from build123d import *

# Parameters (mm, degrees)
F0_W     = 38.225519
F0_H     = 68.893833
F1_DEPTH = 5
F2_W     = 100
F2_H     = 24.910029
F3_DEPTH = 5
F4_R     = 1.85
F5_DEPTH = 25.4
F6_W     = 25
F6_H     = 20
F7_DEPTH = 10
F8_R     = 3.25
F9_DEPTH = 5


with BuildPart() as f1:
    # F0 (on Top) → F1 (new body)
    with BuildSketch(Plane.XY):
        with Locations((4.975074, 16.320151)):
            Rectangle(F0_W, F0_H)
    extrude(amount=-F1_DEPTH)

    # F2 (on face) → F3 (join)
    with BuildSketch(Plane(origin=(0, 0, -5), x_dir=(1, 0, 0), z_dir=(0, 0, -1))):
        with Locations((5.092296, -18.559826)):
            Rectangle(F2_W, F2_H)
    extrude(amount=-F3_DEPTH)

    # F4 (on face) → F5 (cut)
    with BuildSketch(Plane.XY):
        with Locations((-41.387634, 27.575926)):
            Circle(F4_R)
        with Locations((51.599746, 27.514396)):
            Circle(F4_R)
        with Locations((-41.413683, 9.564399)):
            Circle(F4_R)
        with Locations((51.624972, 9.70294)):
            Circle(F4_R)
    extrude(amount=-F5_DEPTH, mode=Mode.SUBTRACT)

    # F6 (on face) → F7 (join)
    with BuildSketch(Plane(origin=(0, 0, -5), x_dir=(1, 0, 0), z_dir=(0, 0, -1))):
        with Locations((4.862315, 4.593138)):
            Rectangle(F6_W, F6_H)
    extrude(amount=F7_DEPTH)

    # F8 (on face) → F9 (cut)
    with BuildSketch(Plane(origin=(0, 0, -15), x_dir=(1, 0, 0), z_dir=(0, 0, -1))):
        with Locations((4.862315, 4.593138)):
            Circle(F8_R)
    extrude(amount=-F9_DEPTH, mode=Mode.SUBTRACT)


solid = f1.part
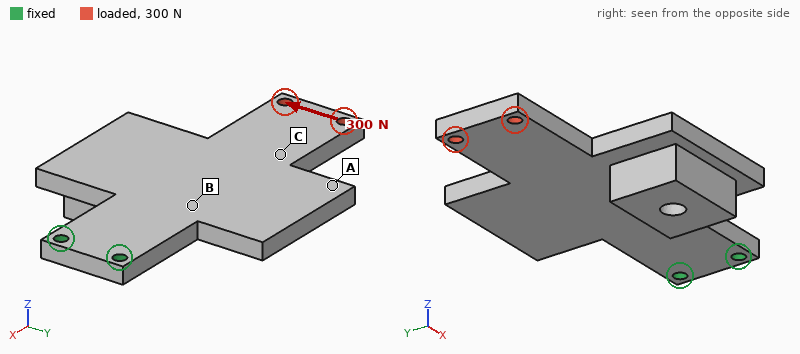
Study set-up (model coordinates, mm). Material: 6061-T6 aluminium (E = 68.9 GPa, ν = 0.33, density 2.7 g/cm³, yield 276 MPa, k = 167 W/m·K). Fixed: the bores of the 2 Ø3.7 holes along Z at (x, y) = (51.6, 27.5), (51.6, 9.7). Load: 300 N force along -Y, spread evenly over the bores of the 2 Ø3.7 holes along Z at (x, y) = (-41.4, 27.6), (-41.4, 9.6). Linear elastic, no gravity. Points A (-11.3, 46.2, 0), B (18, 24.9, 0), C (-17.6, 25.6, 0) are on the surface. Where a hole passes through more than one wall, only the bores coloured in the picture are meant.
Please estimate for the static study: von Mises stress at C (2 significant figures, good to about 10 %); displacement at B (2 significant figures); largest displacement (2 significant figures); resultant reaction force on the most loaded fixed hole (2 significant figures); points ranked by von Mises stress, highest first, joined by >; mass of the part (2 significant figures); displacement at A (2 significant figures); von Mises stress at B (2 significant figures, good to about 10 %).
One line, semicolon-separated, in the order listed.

7.7 MPa; 0.036 mm; 0.17 mm; 1.5 kN; B > C > A; 69 g; 0.10 mm; 16 MPa
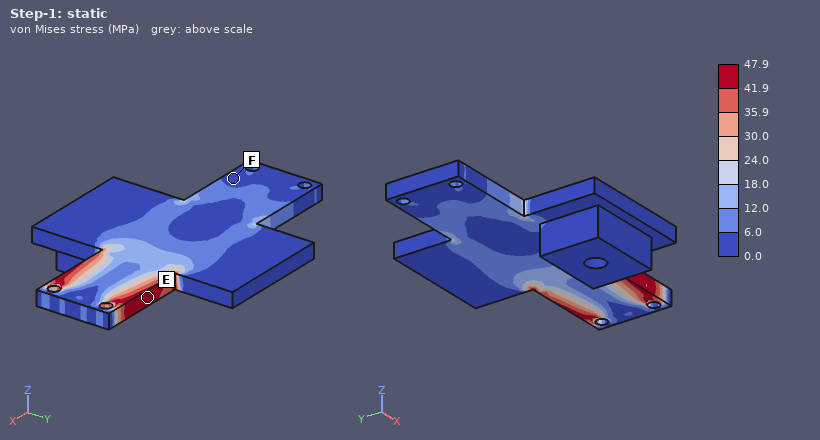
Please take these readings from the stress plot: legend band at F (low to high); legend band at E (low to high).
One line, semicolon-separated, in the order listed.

0.0 to 6.0 MPa; 41.9 to 47.9 MPa
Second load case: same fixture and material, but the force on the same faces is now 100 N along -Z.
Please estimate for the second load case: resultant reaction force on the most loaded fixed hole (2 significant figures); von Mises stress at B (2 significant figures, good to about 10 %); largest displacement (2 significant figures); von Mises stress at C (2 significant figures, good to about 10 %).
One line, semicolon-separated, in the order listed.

50 N; 38 MPa; 1.4 mm; 23 MPa
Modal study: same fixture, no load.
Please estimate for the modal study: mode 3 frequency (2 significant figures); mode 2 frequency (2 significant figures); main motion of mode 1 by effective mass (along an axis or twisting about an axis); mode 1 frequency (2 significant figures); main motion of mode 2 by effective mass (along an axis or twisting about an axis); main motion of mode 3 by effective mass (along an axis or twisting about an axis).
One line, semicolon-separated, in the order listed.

1600 Hz; 970 Hz; along Z; 370 Hz; twisting about X; along Y
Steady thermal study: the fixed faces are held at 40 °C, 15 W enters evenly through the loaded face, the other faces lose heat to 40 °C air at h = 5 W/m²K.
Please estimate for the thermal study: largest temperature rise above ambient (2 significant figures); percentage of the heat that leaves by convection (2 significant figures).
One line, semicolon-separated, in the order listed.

56 K; 9.5 %
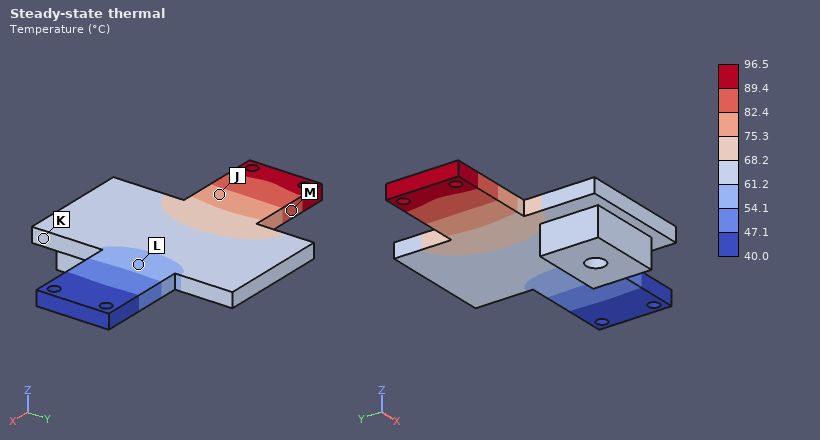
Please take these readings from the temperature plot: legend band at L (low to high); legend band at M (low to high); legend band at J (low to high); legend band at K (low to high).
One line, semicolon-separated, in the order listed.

54.1 to 61.2 °C; 82.4 to 89.4 °C; 75.3 to 82.4 °C; 61.2 to 68.2 °C
